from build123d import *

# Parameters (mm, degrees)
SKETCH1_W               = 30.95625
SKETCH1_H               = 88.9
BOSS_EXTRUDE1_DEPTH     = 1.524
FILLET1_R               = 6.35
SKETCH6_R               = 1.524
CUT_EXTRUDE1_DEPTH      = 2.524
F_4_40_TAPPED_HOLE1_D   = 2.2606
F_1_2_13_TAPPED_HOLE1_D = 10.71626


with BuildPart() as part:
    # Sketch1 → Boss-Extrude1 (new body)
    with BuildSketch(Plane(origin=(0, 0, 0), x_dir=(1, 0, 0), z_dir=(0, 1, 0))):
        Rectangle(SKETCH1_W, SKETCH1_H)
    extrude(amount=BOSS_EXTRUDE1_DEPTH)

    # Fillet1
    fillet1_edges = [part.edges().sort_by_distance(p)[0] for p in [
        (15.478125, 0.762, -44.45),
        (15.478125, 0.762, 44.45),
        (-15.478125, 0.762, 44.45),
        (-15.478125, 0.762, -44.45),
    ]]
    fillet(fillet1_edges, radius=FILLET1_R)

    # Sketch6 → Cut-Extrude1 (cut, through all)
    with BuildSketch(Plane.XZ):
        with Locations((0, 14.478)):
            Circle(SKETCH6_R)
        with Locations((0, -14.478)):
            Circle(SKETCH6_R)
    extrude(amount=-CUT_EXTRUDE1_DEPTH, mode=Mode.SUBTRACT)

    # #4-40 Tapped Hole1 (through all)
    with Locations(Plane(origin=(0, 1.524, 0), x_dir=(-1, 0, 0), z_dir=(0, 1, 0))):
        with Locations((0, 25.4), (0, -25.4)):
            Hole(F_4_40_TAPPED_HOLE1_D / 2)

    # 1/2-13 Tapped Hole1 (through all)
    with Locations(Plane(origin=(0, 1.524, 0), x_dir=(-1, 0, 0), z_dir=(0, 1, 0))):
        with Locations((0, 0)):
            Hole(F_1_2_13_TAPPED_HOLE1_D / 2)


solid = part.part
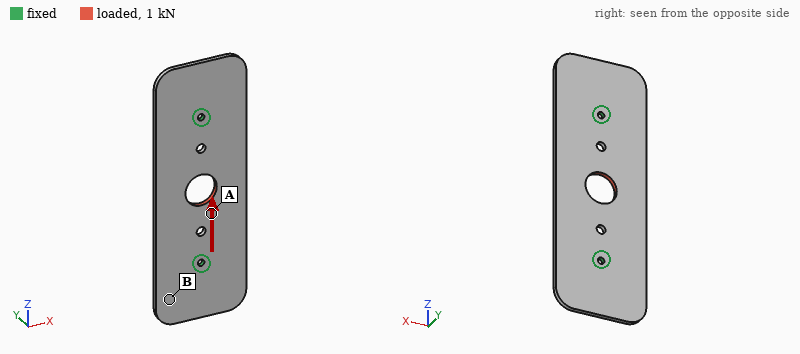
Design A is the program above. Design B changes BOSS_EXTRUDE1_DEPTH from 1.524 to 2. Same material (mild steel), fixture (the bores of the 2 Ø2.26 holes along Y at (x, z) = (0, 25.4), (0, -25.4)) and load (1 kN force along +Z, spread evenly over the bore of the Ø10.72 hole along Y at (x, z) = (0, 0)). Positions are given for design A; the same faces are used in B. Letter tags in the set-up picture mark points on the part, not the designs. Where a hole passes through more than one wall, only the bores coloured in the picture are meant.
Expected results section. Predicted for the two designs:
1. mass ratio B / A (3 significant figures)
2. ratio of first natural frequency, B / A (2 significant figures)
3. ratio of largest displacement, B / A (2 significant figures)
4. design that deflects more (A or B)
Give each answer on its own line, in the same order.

1.31
1.3
0.76
A
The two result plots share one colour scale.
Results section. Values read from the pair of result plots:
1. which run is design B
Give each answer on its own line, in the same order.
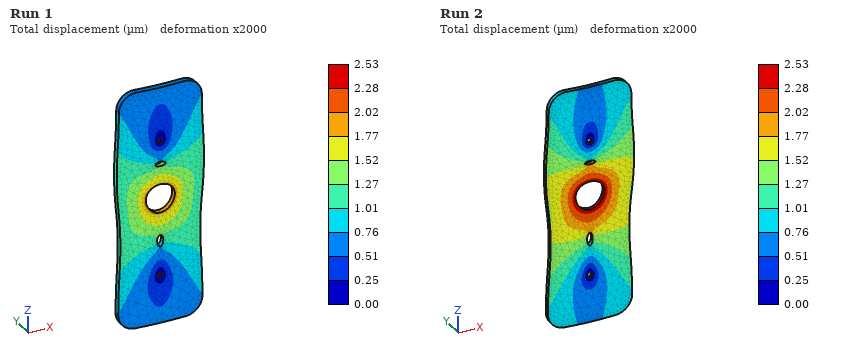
Run 1
